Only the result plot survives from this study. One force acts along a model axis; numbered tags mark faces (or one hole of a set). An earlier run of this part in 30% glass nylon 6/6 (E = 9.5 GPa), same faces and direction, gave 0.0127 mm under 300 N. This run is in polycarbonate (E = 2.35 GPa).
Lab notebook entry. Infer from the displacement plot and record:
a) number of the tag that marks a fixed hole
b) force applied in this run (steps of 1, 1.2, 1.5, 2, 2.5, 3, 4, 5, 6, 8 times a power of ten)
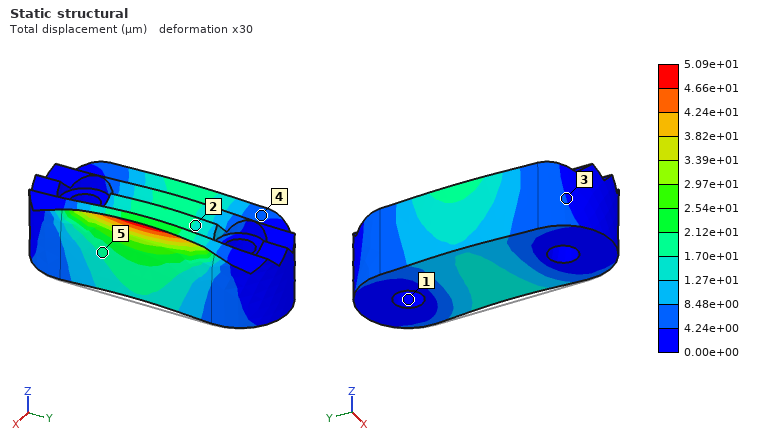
1
300 N
